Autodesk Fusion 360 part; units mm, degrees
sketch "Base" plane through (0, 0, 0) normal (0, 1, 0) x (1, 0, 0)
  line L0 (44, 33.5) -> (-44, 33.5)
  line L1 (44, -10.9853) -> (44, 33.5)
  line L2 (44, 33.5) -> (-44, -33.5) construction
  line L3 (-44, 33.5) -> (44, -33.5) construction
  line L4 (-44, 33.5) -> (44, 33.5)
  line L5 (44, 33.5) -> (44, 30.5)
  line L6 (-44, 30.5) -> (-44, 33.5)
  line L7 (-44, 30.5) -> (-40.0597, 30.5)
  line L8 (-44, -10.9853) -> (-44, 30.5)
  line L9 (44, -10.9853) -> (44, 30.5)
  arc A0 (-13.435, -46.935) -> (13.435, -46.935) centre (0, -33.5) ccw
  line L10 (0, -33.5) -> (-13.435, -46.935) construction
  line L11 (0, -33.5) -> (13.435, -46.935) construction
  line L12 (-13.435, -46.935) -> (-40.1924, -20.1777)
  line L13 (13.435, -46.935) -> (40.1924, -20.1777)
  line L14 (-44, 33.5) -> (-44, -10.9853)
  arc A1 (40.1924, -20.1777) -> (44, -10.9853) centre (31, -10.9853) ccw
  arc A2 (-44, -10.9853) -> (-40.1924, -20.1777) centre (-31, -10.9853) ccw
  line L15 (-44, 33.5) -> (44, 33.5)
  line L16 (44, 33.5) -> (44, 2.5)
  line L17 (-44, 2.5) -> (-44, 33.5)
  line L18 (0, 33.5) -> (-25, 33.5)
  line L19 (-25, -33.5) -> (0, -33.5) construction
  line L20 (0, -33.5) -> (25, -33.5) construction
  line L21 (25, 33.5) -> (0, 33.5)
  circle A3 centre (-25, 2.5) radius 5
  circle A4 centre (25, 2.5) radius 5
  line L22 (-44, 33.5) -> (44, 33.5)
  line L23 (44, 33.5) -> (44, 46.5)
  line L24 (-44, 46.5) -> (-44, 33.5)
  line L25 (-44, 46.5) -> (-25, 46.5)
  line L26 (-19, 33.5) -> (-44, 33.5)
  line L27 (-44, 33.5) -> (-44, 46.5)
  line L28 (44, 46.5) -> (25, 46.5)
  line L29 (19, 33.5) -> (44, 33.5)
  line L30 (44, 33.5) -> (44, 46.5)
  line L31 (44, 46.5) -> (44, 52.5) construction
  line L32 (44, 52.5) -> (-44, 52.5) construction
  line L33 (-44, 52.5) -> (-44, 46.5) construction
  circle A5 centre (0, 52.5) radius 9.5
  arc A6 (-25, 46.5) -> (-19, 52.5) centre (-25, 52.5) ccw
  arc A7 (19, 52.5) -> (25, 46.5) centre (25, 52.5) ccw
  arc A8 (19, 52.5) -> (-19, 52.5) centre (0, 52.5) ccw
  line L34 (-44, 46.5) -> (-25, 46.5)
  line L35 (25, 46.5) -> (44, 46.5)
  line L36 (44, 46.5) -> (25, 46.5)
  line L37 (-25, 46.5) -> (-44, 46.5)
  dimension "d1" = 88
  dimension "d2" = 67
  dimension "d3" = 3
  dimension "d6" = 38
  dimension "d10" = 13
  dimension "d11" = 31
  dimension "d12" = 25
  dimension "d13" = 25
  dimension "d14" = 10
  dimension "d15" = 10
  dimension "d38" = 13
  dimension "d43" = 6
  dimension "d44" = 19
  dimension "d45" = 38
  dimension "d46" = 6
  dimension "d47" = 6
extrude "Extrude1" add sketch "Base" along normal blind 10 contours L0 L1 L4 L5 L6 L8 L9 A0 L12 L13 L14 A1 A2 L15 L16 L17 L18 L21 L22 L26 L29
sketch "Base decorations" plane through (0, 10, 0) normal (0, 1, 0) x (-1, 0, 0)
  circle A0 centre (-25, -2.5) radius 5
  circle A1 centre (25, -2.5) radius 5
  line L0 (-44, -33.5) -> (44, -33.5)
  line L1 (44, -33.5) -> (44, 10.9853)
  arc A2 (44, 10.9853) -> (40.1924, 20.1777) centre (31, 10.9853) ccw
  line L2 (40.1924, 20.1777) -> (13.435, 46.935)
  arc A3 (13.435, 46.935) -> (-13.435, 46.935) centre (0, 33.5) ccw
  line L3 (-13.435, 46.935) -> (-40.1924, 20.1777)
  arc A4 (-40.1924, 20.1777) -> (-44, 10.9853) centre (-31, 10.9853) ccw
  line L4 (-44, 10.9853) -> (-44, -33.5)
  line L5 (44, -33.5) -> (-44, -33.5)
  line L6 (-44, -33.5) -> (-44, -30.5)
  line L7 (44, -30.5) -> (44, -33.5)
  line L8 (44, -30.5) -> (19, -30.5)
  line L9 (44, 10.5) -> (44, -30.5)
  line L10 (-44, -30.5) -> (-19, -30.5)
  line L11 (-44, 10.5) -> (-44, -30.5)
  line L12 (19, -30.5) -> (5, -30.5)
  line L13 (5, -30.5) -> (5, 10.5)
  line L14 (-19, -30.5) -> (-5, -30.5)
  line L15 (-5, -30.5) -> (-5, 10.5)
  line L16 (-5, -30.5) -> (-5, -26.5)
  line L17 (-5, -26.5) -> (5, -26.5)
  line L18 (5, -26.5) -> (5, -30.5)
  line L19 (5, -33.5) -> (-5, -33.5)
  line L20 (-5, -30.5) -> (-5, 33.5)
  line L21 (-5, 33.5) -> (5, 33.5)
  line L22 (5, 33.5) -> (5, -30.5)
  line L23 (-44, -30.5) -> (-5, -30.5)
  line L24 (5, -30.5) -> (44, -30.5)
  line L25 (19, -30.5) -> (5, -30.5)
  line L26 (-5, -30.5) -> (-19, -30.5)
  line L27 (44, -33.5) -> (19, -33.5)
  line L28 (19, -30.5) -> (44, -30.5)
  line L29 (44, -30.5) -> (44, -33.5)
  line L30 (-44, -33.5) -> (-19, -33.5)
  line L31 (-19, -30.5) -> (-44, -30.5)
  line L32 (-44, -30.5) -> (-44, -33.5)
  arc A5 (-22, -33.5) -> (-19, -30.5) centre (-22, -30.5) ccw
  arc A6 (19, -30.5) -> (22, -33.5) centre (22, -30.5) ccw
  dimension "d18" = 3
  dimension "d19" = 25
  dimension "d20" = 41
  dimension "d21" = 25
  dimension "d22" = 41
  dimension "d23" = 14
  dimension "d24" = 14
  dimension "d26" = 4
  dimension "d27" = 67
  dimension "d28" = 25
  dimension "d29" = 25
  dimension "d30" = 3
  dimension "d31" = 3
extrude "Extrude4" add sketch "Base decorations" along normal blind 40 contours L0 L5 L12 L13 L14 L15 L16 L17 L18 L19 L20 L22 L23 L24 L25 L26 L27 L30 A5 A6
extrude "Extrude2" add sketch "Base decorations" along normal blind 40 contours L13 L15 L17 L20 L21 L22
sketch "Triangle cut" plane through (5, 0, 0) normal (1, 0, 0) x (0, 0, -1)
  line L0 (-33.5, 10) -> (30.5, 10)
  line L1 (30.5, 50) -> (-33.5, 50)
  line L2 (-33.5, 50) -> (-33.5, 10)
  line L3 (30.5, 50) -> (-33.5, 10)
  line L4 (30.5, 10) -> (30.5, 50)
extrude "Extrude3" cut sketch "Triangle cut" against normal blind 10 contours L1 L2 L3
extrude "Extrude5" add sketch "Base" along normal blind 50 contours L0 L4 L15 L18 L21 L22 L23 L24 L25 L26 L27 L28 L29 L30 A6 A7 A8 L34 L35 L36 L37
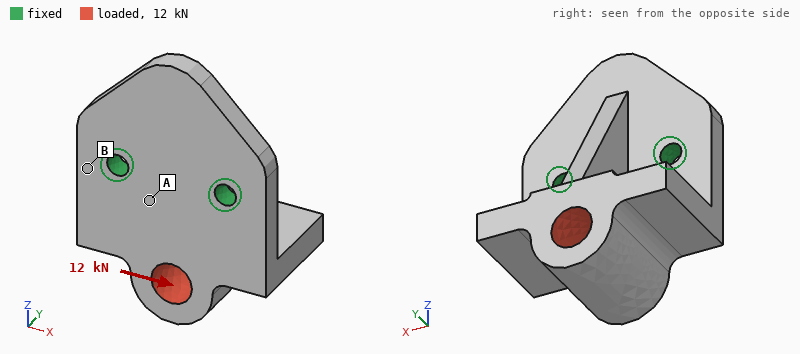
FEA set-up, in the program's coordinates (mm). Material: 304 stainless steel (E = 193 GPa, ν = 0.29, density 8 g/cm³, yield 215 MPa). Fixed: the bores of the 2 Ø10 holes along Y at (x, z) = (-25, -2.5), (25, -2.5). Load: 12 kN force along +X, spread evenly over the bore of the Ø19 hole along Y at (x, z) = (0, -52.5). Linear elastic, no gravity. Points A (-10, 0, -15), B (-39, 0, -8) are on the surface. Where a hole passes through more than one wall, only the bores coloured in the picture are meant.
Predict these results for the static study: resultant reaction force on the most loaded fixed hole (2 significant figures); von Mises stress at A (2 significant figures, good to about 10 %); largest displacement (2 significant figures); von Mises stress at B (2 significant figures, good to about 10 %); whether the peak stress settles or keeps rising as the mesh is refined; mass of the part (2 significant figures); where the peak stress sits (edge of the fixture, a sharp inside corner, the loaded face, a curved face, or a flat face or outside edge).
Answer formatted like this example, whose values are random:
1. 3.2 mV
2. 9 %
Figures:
1. 13 kN
2. 16 MPa
3. 61 µm
4. 68 MPa
5. keeps rising
6. 1.3 kg
7. edge of the fixture
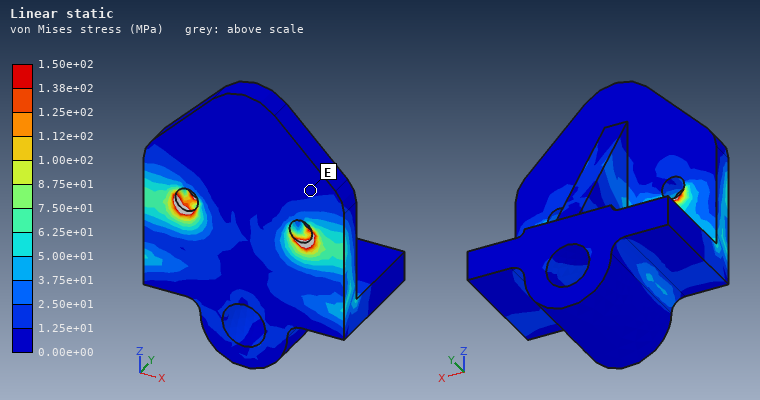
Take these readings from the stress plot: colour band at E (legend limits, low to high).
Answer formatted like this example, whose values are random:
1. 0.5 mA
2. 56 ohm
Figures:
1. 0.00e+00 to 1.25e+01 MPa
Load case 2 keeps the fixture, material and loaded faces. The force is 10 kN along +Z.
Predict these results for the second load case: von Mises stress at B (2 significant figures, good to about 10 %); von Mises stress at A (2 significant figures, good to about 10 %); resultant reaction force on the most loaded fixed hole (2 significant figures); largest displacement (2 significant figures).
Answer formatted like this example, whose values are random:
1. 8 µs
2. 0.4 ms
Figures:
1. 36 MPa
2. 24 MPa
3. 5.0 kN
4. 0.10 mm
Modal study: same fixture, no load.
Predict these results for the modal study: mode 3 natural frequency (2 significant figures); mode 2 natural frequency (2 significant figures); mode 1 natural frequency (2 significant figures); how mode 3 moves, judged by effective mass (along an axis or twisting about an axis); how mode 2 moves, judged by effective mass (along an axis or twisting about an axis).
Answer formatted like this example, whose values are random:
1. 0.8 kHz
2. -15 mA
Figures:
1. 5100 Hz
2. 2800 Hz
3. 1500 Hz
4. along Y
5. along X
